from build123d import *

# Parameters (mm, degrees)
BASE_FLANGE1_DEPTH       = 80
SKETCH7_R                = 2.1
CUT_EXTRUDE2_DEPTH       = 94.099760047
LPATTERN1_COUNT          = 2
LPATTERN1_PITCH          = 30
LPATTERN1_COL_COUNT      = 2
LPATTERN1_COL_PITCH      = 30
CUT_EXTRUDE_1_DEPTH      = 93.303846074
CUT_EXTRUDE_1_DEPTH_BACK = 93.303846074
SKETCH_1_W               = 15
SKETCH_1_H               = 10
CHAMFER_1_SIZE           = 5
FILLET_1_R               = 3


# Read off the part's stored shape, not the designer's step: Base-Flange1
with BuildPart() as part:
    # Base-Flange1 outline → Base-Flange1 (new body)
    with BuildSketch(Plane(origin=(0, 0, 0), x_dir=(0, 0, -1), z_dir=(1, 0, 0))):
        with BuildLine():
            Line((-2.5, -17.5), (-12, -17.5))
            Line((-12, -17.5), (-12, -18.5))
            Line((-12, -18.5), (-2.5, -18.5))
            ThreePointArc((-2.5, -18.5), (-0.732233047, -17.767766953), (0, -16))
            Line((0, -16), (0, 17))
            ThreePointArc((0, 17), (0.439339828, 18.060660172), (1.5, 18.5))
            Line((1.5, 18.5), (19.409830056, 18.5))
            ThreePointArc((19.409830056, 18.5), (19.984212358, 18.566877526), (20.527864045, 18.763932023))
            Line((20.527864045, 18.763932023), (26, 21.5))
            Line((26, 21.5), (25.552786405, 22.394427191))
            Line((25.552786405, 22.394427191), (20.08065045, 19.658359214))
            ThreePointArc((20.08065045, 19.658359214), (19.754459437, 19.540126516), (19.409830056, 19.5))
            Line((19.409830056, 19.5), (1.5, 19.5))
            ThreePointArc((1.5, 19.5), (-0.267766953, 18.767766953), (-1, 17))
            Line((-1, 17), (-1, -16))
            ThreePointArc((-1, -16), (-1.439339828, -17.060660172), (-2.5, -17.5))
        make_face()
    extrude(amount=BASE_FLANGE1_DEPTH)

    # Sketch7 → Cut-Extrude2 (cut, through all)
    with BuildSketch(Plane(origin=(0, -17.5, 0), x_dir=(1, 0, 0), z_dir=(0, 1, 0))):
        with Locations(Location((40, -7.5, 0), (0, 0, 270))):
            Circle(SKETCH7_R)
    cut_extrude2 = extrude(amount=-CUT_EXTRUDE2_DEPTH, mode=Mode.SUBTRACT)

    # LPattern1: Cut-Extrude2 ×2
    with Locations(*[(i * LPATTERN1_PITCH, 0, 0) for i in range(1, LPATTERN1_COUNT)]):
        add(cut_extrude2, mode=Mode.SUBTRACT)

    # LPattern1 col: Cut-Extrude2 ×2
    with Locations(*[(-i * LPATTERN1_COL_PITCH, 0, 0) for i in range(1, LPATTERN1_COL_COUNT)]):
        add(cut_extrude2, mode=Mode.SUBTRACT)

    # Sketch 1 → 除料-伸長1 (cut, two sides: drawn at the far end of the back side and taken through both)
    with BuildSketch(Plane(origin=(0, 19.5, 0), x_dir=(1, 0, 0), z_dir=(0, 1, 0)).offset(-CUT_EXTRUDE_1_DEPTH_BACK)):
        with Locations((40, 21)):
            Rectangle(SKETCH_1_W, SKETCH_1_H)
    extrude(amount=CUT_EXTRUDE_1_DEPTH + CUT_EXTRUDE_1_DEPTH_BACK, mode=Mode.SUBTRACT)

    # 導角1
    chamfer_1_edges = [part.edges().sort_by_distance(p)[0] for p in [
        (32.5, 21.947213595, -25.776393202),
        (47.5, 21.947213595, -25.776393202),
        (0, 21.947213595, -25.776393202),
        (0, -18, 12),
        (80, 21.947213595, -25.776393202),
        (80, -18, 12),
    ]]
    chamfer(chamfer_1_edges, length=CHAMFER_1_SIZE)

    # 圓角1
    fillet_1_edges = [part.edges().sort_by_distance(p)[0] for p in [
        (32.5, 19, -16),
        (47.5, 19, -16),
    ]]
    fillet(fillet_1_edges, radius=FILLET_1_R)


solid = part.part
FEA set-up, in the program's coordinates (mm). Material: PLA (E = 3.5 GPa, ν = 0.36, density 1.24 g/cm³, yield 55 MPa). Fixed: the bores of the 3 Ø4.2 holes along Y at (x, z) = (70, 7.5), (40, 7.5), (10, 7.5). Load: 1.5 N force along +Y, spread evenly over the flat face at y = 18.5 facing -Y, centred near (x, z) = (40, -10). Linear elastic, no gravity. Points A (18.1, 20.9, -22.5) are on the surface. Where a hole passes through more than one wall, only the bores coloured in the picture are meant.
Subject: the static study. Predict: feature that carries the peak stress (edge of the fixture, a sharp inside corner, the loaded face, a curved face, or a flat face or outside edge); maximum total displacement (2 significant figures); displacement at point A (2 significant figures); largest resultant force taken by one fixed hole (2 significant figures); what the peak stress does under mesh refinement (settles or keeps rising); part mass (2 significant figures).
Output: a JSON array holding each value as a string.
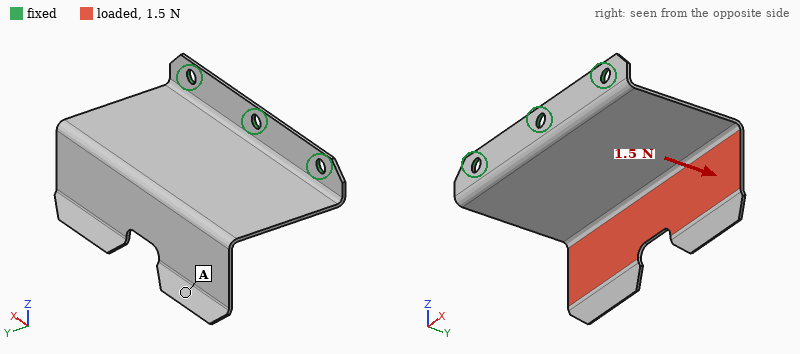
["edge of the fixture", "1.1 mm", "0.99 mm", "0.57 N", "keeps rising", "7.0 g"]
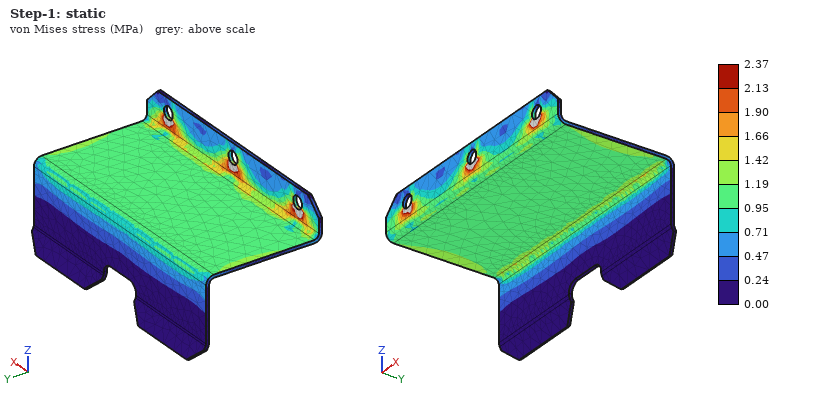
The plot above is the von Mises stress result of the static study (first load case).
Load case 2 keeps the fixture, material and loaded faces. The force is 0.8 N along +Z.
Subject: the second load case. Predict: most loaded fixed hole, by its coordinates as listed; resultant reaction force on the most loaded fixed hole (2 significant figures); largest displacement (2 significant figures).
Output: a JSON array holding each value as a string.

["(40, 7.5)", "0.46 N", "1.1 mm"]
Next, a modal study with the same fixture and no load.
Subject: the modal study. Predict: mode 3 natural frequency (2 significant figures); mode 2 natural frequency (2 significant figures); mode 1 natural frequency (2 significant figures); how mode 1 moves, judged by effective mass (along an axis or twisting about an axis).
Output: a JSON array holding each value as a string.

["300 Hz", "140 Hz", "79 Hz", "along Z"]
